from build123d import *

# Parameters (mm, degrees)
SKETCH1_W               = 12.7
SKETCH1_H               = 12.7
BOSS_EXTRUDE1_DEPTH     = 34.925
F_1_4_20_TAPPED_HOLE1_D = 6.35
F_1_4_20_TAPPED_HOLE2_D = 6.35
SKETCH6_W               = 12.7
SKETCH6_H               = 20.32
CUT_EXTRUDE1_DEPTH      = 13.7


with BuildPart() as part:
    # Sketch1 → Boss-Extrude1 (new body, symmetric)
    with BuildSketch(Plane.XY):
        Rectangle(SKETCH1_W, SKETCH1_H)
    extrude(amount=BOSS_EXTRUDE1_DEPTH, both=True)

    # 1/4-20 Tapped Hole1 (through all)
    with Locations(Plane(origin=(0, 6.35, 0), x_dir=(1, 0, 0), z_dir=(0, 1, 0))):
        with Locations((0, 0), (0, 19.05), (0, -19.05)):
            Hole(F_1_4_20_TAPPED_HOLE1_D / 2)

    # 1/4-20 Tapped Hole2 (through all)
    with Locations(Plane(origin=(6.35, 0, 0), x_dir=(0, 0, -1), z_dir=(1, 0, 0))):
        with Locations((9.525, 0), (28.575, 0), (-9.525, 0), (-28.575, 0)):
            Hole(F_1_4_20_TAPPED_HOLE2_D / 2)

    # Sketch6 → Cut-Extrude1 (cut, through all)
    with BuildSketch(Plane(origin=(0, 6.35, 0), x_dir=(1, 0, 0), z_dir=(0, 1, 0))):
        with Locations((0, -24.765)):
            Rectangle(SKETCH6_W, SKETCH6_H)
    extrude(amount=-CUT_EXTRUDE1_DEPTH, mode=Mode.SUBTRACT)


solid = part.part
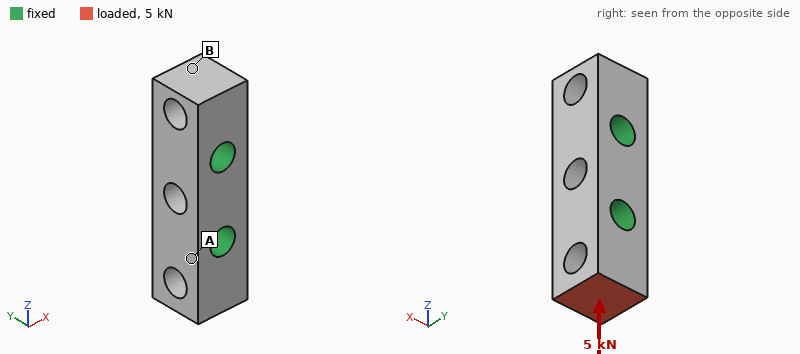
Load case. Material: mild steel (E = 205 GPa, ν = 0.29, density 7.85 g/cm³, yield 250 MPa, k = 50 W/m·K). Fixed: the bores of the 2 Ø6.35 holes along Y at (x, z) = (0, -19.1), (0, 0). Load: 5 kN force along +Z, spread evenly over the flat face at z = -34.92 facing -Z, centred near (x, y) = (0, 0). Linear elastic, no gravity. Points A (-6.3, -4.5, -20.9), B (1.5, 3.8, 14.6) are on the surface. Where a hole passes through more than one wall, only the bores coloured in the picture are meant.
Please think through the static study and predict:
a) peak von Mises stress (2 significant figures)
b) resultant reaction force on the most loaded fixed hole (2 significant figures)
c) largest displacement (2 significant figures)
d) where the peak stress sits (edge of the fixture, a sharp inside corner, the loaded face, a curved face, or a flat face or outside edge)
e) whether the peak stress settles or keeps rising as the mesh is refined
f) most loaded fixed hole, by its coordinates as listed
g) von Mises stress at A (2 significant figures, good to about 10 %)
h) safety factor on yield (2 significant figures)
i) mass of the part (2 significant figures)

150 MPa
4.9 kN
5.3 µm
a curved face
settles
(0, -19.1)
27 MPa
1.6
47 g
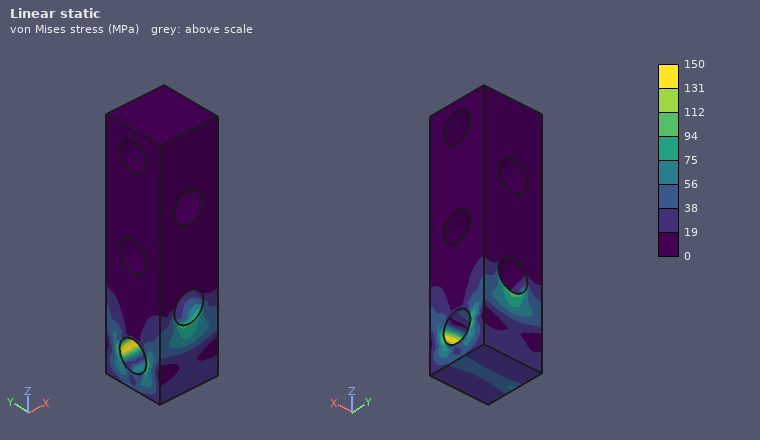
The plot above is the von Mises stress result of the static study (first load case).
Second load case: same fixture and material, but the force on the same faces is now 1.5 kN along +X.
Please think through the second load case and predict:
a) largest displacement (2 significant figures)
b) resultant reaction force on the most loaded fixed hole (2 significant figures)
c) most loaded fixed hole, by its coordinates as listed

11 µm
1.7 kN
(0, -19.1)
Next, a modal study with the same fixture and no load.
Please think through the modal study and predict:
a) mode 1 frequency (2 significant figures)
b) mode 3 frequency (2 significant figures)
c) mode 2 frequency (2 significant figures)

29 kHz
34 kHz
30 kHz
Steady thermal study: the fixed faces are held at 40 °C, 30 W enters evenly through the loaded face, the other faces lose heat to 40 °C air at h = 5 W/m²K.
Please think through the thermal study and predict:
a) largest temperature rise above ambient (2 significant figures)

77 K
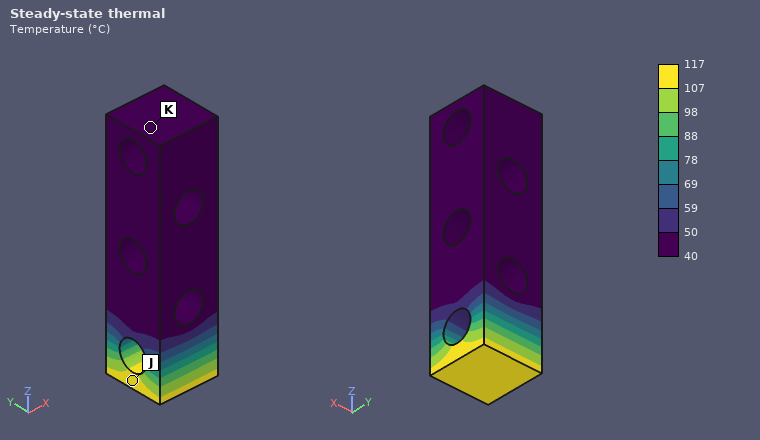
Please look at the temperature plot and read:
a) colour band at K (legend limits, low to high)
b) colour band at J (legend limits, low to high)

40 to 50 °C
107 to 117 °C
